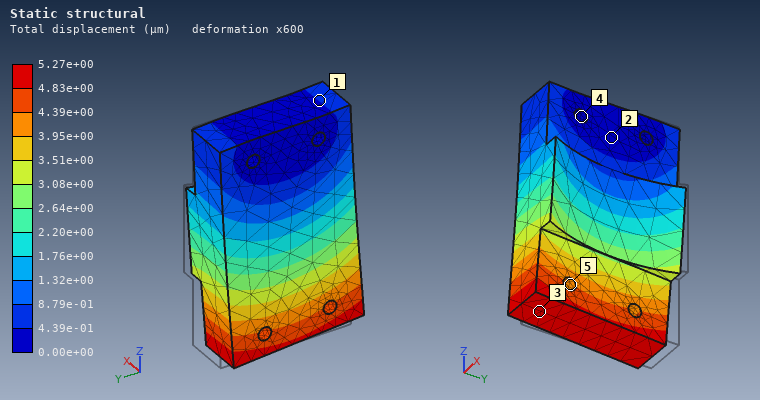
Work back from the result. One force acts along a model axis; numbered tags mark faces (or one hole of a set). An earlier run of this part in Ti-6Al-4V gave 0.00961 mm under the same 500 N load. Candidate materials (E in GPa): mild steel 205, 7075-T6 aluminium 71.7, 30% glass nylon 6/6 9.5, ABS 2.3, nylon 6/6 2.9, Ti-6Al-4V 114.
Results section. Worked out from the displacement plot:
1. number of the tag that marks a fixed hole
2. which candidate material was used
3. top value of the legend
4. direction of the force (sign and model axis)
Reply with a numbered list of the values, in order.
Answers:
1. 4
2. mild steel
3. 5.27e+00 µm
4. -Y
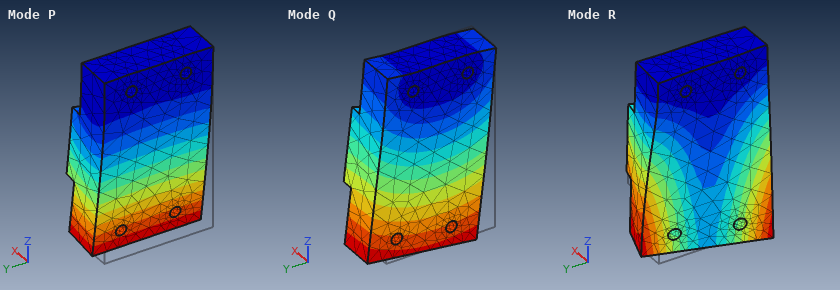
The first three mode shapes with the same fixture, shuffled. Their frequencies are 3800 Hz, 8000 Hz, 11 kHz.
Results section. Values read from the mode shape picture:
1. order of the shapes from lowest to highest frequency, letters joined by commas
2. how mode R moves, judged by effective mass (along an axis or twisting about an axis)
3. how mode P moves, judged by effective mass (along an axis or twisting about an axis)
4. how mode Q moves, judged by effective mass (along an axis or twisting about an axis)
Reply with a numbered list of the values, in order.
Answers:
1. P, Q, R
2. twisting about Z
3. along X
4. along Y
